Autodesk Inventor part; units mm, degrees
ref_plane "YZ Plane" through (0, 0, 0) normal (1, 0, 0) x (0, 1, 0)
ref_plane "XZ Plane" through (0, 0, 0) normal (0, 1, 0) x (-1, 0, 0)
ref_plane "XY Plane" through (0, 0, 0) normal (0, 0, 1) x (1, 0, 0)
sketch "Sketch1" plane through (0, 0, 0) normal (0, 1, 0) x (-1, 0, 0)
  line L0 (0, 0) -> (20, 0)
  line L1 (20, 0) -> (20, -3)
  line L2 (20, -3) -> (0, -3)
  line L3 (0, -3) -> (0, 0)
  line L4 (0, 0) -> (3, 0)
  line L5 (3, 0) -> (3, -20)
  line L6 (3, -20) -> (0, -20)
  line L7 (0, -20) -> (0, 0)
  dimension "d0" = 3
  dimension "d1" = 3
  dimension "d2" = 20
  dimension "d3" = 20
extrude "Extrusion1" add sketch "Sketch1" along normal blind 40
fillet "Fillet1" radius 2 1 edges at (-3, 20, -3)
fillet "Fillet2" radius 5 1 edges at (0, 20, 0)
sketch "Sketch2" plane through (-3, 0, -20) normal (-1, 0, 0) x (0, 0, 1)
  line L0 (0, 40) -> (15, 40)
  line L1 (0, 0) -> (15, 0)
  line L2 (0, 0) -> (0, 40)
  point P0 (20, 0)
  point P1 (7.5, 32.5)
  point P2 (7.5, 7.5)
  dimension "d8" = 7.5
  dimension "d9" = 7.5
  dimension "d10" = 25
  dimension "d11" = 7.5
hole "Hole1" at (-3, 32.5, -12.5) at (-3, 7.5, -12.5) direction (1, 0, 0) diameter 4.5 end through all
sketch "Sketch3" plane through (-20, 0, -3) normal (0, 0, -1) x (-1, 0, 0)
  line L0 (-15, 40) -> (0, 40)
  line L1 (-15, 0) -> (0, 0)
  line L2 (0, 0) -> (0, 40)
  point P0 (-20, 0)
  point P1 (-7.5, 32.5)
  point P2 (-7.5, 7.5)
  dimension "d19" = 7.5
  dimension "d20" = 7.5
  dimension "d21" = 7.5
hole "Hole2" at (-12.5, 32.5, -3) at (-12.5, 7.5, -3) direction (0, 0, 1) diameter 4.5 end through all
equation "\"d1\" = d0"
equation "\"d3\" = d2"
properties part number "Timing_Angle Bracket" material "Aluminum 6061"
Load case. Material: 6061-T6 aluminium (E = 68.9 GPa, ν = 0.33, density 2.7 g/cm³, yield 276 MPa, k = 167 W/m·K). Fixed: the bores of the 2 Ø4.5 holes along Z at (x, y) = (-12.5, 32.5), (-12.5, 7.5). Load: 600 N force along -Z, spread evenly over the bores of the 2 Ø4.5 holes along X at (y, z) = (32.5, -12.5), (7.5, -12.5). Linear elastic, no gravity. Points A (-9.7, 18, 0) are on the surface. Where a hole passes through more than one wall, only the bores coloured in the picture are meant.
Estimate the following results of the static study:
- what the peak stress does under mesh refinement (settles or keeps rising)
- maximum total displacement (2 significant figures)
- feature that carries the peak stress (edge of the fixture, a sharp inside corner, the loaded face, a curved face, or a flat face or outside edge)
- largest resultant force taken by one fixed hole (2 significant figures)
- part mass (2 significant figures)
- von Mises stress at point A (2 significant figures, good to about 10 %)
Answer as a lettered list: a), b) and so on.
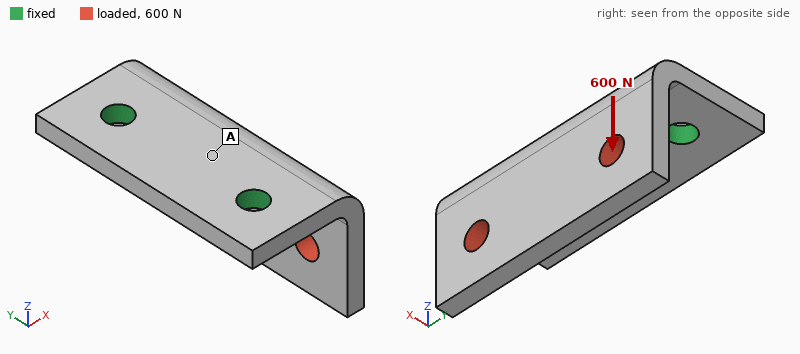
a) keeps rising
b) 0.11 mm
c) edge of the fixture
d) 300 N
e) 11 g
f) 33 MPa
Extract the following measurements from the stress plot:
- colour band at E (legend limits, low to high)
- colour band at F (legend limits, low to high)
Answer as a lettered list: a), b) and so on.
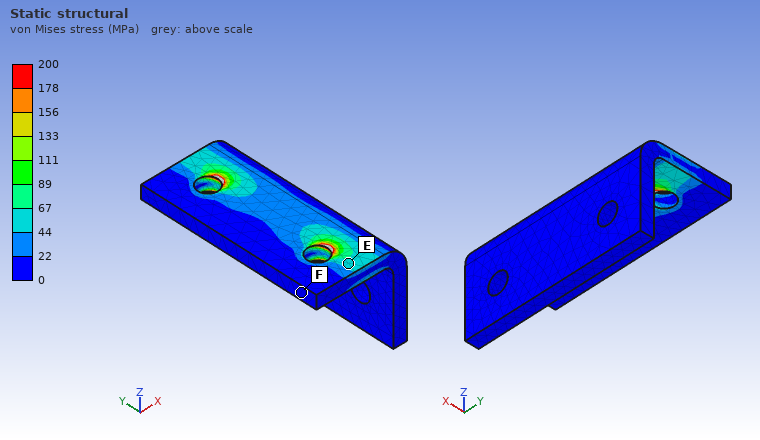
a) 44 to 67 MPa
b) 0 to 22 MPa
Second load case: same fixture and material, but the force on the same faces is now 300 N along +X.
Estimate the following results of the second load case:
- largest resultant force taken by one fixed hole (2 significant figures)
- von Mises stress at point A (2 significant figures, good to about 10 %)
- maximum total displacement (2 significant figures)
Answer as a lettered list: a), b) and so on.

a) 150 N
b) 30 MPa
c) 0.13 mm
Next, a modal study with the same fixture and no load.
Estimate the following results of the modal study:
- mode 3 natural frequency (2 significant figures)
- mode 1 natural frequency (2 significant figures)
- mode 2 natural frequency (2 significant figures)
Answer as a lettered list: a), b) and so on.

a) 12 kHz
b) 4000 Hz
c) 6800 Hz
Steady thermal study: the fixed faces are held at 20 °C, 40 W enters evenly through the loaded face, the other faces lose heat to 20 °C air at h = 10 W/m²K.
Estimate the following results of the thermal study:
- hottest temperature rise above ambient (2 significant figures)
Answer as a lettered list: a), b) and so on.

a) 50 K
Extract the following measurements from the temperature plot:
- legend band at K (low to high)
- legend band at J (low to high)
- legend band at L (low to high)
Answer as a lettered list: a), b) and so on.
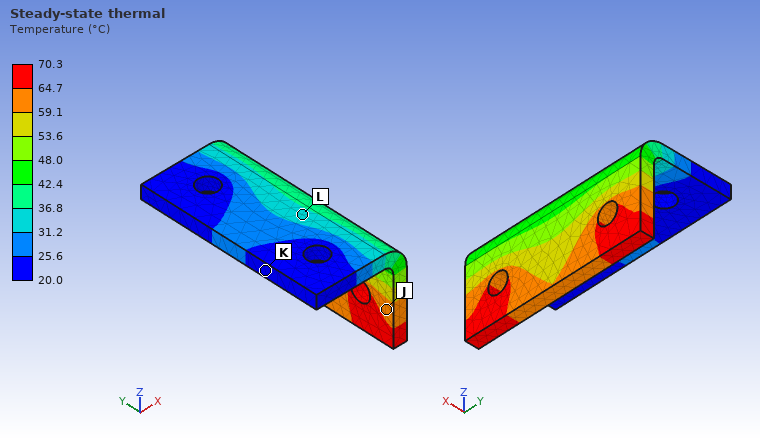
a) 20.0 to 25.6 °C
b) 59.1 to 64.7 °C
c) 31.2 to 36.8 °C
